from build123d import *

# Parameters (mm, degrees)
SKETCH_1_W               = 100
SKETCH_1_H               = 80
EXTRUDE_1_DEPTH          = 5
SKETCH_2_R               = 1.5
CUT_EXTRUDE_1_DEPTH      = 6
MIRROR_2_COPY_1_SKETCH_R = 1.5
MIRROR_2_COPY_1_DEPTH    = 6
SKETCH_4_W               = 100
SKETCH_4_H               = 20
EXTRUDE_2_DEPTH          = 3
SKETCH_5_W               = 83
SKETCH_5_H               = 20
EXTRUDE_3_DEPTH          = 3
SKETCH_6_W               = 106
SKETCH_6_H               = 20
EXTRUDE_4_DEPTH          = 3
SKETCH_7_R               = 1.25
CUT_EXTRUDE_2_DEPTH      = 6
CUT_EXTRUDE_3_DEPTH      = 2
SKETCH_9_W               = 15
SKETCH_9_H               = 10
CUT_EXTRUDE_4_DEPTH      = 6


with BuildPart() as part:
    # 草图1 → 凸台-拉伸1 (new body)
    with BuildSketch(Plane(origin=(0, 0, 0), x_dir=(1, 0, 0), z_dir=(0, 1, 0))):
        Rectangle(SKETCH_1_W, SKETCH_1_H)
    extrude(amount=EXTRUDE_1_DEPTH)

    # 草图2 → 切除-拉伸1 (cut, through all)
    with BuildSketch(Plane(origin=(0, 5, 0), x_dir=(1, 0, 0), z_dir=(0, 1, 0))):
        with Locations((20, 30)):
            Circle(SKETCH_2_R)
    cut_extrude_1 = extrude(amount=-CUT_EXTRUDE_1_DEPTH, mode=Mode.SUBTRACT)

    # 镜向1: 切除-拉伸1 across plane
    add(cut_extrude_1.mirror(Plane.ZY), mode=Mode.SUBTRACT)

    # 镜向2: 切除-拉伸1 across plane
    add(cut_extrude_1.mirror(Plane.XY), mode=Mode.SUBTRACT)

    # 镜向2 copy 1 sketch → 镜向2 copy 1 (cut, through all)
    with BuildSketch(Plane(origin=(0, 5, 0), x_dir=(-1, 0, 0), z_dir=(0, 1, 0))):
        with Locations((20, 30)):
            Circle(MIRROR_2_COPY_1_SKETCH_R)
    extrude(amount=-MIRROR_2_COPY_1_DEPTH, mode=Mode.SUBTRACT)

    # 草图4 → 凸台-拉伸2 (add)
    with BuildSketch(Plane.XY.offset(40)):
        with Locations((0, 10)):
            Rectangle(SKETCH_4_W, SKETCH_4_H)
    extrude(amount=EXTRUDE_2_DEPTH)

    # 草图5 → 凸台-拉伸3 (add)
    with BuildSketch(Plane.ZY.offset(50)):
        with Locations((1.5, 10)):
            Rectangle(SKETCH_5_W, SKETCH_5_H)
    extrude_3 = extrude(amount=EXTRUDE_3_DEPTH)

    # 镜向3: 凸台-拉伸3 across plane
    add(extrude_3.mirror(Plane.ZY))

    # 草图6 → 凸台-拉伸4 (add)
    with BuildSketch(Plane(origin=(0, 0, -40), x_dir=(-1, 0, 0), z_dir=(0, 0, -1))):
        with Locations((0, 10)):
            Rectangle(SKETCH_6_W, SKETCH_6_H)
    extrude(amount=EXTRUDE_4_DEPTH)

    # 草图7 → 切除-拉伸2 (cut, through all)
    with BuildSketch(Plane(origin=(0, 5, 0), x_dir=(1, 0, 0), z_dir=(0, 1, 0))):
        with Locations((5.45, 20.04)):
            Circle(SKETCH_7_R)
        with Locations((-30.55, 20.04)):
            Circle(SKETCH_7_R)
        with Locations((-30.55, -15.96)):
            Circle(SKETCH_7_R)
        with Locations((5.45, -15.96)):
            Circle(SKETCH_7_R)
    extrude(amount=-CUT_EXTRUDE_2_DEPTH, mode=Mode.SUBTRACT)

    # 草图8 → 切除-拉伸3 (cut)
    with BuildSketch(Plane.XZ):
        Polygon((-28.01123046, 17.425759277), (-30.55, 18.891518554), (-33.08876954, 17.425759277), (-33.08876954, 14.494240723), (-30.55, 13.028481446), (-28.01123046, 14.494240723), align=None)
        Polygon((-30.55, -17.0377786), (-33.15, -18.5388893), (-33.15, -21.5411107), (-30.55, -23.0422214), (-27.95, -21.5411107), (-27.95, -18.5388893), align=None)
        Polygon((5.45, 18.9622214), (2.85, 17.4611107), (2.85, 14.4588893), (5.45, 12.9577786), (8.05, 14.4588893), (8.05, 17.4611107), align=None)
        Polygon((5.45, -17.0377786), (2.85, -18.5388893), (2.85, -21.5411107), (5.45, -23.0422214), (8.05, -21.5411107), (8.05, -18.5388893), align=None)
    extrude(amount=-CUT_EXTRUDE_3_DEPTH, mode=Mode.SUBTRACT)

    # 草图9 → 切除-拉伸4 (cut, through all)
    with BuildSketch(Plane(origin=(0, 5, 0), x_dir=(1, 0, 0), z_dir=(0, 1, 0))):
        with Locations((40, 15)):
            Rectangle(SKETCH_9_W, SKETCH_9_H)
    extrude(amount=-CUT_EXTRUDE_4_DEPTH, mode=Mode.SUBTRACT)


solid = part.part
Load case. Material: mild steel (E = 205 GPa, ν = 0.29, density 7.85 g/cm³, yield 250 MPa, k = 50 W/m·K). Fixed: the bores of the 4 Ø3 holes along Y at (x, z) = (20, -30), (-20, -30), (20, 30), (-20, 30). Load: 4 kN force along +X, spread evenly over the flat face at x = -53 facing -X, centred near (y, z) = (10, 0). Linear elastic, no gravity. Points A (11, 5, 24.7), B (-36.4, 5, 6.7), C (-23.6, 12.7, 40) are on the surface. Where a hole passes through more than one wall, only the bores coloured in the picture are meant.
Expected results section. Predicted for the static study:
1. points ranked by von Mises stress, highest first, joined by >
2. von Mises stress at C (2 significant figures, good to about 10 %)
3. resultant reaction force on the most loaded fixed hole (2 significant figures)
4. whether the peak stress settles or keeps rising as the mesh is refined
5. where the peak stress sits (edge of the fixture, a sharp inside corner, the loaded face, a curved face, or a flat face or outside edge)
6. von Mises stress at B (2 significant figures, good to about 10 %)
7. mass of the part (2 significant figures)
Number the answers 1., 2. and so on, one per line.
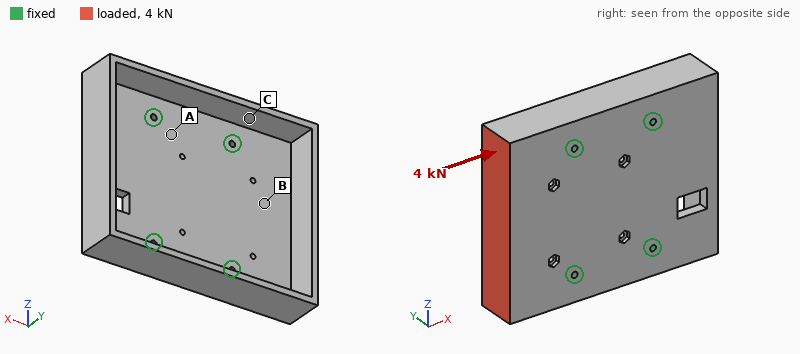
1. B > C > A
2. 20 MPa
3. 1.3 kN
4. keeps rising
5. edge of the fixture
6. 42 MPa
7. 480 g
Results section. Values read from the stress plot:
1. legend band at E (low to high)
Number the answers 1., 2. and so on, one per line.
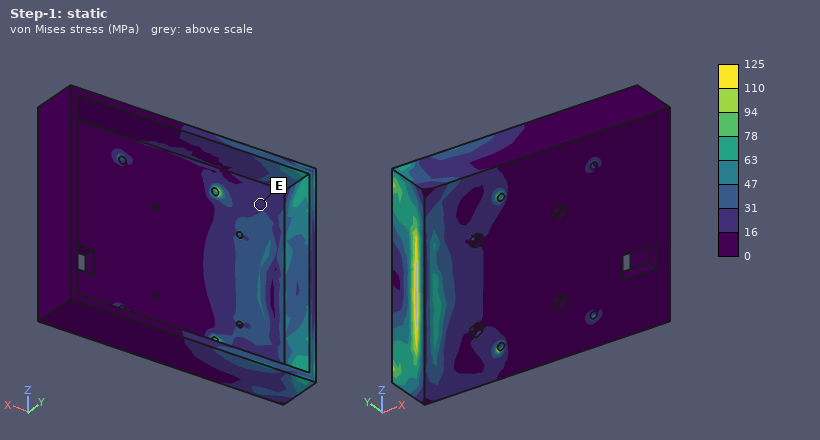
1. 16 to 31 MPa
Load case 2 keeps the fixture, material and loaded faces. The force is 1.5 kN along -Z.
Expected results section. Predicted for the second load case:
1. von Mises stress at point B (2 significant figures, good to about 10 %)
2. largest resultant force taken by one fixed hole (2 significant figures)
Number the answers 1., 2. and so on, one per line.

1. 14 MPa
2. 1.0 kN
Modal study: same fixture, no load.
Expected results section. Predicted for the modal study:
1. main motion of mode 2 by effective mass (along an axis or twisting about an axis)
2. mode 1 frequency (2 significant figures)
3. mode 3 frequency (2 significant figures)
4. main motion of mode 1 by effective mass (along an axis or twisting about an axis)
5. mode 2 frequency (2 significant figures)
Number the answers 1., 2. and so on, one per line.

1. along Y
2. 3200 Hz
3. 4100 Hz
4. twisting about Z
5. 3700 Hz
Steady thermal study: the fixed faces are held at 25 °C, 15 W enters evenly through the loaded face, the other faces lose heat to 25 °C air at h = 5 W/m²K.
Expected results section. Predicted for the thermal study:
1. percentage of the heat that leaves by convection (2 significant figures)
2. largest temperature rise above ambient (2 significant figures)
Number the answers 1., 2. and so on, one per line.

1. 7.1 %
2. 32 K
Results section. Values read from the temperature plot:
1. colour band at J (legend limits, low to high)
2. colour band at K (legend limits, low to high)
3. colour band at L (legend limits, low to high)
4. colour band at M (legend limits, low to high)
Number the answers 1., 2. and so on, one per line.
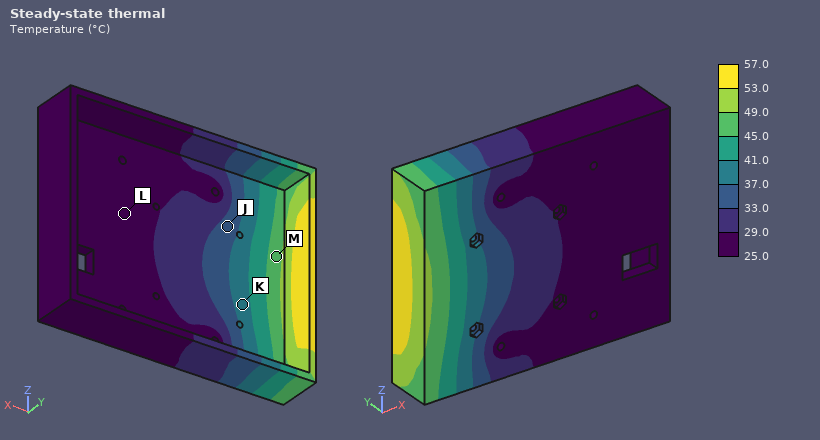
1. 33.0 to 37.0 °C
2. 37.0 to 41.0 °C
3. 25.0 to 29.0 °C
4. 45.0 to 49.0 °C
